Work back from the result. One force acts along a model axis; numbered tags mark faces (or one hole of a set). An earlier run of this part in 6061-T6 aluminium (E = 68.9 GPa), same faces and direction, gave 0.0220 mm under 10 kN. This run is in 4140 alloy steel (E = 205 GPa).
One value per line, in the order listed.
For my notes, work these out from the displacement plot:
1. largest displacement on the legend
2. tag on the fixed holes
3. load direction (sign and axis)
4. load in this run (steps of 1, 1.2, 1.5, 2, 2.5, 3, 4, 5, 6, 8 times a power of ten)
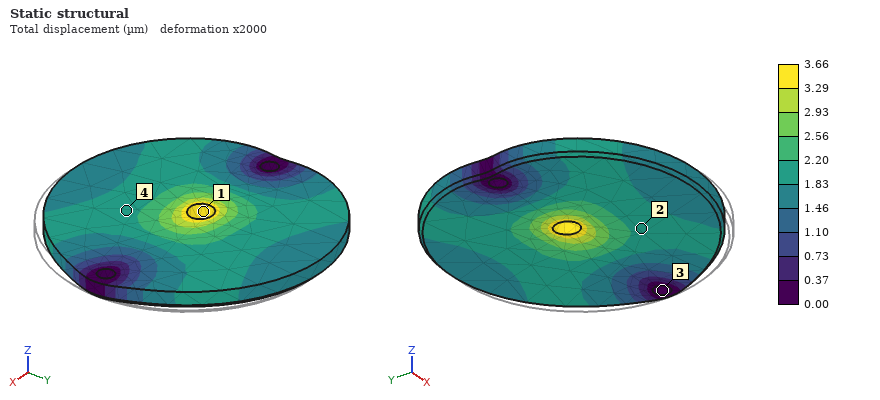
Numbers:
3.66 µm
3
-X
5 kN
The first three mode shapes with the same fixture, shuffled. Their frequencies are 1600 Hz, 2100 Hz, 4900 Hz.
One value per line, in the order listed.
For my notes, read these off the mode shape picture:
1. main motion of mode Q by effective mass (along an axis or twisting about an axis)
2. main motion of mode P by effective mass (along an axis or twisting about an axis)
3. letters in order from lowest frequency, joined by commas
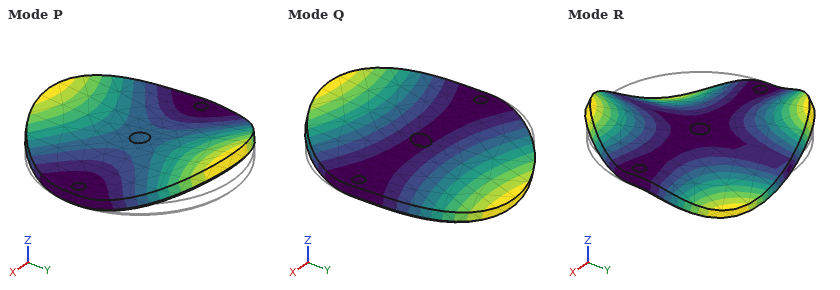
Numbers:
twisting about X
along Z
Q, P, R
